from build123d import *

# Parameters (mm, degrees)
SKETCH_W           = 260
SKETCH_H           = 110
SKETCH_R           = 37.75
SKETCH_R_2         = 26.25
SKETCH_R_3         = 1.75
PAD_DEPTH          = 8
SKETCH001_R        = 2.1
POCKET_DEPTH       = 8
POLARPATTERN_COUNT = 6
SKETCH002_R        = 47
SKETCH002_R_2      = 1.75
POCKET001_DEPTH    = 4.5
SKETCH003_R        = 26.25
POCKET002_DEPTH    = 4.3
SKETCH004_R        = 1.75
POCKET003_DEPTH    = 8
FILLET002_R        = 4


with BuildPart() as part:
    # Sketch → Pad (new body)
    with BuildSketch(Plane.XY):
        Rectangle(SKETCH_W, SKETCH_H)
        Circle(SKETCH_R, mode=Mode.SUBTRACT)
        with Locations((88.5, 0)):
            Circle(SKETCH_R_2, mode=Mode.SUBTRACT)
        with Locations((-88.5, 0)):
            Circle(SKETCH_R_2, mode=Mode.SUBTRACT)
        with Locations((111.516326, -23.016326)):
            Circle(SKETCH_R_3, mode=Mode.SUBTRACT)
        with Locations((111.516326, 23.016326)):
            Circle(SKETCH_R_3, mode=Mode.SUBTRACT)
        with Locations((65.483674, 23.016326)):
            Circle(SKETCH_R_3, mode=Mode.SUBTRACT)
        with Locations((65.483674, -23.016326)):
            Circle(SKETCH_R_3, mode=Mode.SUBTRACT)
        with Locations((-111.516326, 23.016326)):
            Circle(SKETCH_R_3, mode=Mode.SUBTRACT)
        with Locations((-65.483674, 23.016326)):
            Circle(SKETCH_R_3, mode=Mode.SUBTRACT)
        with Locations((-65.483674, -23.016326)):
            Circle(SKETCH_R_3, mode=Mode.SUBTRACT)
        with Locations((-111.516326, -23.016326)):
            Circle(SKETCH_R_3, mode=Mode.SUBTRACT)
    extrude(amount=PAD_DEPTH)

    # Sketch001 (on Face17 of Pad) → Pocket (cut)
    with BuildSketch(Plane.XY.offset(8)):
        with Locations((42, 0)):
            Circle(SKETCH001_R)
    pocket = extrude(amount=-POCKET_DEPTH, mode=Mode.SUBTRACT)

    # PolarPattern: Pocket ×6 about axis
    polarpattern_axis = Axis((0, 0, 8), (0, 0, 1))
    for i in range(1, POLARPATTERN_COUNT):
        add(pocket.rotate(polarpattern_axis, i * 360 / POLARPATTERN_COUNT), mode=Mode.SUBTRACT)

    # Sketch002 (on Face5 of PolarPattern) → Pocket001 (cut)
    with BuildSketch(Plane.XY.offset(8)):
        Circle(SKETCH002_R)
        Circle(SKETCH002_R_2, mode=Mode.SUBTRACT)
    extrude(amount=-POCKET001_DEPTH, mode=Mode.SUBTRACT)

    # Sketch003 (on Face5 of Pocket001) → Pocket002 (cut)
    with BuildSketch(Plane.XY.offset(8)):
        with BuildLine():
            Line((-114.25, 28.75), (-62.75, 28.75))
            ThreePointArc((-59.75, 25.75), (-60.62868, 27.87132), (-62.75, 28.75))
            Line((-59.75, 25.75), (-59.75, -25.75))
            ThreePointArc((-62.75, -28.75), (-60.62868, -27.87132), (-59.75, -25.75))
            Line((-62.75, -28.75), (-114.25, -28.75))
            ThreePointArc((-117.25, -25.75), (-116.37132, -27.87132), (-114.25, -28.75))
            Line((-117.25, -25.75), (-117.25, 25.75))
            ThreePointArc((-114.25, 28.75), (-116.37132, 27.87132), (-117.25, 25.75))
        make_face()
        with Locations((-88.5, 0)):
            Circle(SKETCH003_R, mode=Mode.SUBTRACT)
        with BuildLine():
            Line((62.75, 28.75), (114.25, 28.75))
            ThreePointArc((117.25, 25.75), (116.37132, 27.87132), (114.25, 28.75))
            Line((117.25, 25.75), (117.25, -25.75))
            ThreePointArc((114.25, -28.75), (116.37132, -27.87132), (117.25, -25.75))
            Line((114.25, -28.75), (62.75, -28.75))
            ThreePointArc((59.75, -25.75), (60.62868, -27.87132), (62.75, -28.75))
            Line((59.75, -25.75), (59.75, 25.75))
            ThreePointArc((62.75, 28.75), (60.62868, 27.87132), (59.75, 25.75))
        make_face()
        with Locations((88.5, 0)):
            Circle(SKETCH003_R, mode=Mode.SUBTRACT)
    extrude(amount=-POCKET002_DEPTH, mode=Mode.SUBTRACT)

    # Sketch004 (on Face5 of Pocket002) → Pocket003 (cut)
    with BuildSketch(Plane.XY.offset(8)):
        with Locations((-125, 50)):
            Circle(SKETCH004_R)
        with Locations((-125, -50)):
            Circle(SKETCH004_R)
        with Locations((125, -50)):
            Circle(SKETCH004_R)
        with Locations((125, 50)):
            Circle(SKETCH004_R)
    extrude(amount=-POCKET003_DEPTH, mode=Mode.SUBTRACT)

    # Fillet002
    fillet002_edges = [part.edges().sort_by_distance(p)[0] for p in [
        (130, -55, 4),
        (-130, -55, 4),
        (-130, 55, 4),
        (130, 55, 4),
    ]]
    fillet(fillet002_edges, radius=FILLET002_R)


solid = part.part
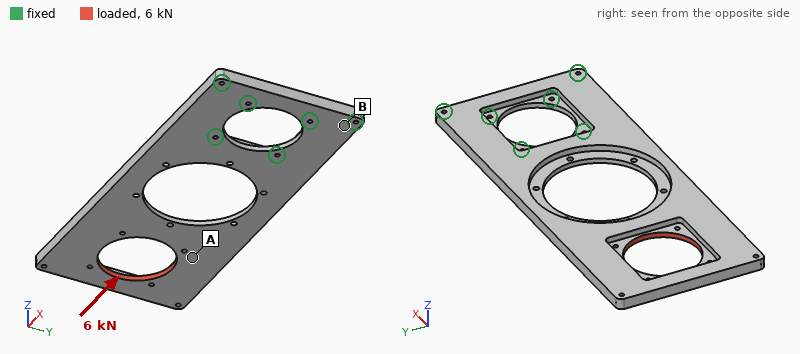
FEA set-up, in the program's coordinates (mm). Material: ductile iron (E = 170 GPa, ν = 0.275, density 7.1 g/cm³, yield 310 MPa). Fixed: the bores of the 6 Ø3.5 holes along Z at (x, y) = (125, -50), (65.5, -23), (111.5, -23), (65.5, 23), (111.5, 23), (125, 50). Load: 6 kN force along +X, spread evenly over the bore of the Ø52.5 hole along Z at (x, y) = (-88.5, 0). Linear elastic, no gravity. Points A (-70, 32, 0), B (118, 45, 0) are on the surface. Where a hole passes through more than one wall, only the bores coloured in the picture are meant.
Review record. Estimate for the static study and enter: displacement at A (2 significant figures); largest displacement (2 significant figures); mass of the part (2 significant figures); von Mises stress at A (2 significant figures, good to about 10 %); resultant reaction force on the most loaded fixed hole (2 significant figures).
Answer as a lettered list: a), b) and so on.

a) 0.33 mm
b) 0.64 mm
c) 970 g
d) 21 MPa
e) 1.5 kN
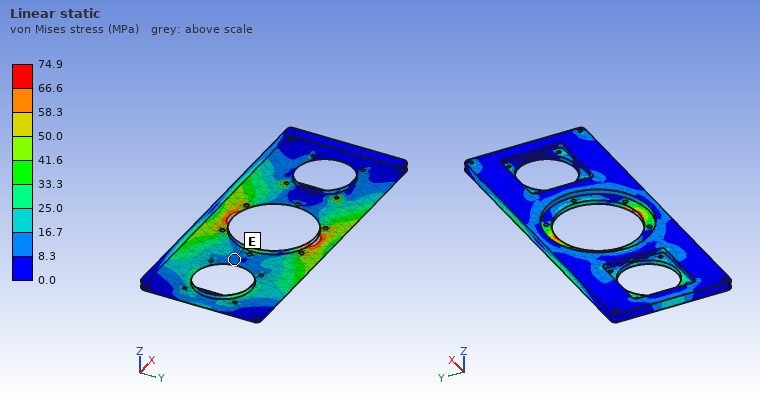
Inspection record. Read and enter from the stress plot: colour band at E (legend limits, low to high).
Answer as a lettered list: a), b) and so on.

a) 8.3 to 16.7 MPa
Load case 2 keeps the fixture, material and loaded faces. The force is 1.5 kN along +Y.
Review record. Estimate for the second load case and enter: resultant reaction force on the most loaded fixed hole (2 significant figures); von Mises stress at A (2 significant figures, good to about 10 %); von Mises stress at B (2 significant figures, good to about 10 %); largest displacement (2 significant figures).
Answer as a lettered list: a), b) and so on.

a) 1.5 kN
b) 10.0 MPa
c) 7.6 MPa
d) 0.11 mm
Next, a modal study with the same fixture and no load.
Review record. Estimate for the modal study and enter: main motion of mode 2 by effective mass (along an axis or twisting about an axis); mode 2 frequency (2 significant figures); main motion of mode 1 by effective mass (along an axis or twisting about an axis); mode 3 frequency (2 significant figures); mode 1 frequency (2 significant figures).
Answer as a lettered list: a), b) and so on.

a) twisting about X
b) 390 Hz
c) along Z
d) 790 Hz
e) 110 Hz
